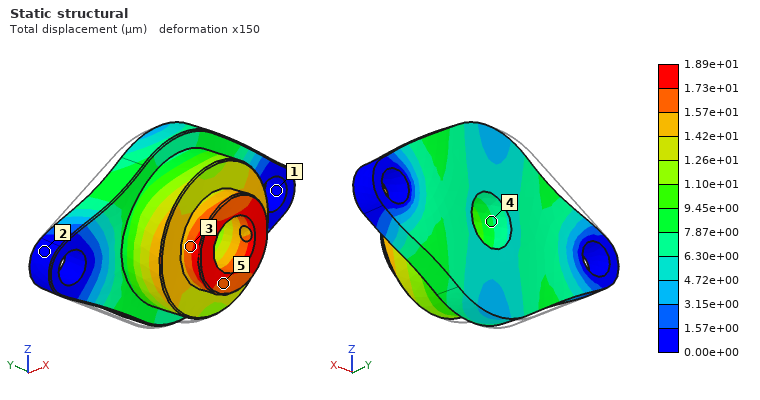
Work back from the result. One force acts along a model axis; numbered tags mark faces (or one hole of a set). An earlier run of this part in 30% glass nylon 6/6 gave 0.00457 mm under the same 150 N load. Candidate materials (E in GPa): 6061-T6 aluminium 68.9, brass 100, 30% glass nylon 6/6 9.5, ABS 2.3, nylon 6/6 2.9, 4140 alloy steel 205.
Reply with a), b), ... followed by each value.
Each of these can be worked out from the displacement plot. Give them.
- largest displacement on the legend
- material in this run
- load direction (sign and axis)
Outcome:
a) 1.89e+01 µm
b) ABS
c) +X
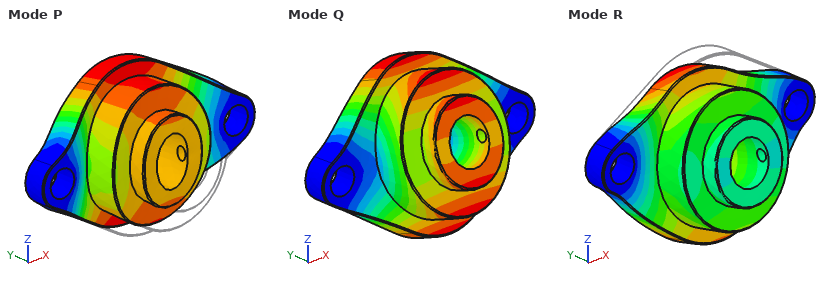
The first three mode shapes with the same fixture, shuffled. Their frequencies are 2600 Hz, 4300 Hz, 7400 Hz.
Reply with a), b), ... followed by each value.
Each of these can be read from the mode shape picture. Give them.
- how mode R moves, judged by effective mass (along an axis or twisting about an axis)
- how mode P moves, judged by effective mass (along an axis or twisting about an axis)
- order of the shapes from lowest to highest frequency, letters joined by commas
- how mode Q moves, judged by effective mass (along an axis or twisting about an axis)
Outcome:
a) along Z
b) along Y
c) Q, P, R
d) along Z
